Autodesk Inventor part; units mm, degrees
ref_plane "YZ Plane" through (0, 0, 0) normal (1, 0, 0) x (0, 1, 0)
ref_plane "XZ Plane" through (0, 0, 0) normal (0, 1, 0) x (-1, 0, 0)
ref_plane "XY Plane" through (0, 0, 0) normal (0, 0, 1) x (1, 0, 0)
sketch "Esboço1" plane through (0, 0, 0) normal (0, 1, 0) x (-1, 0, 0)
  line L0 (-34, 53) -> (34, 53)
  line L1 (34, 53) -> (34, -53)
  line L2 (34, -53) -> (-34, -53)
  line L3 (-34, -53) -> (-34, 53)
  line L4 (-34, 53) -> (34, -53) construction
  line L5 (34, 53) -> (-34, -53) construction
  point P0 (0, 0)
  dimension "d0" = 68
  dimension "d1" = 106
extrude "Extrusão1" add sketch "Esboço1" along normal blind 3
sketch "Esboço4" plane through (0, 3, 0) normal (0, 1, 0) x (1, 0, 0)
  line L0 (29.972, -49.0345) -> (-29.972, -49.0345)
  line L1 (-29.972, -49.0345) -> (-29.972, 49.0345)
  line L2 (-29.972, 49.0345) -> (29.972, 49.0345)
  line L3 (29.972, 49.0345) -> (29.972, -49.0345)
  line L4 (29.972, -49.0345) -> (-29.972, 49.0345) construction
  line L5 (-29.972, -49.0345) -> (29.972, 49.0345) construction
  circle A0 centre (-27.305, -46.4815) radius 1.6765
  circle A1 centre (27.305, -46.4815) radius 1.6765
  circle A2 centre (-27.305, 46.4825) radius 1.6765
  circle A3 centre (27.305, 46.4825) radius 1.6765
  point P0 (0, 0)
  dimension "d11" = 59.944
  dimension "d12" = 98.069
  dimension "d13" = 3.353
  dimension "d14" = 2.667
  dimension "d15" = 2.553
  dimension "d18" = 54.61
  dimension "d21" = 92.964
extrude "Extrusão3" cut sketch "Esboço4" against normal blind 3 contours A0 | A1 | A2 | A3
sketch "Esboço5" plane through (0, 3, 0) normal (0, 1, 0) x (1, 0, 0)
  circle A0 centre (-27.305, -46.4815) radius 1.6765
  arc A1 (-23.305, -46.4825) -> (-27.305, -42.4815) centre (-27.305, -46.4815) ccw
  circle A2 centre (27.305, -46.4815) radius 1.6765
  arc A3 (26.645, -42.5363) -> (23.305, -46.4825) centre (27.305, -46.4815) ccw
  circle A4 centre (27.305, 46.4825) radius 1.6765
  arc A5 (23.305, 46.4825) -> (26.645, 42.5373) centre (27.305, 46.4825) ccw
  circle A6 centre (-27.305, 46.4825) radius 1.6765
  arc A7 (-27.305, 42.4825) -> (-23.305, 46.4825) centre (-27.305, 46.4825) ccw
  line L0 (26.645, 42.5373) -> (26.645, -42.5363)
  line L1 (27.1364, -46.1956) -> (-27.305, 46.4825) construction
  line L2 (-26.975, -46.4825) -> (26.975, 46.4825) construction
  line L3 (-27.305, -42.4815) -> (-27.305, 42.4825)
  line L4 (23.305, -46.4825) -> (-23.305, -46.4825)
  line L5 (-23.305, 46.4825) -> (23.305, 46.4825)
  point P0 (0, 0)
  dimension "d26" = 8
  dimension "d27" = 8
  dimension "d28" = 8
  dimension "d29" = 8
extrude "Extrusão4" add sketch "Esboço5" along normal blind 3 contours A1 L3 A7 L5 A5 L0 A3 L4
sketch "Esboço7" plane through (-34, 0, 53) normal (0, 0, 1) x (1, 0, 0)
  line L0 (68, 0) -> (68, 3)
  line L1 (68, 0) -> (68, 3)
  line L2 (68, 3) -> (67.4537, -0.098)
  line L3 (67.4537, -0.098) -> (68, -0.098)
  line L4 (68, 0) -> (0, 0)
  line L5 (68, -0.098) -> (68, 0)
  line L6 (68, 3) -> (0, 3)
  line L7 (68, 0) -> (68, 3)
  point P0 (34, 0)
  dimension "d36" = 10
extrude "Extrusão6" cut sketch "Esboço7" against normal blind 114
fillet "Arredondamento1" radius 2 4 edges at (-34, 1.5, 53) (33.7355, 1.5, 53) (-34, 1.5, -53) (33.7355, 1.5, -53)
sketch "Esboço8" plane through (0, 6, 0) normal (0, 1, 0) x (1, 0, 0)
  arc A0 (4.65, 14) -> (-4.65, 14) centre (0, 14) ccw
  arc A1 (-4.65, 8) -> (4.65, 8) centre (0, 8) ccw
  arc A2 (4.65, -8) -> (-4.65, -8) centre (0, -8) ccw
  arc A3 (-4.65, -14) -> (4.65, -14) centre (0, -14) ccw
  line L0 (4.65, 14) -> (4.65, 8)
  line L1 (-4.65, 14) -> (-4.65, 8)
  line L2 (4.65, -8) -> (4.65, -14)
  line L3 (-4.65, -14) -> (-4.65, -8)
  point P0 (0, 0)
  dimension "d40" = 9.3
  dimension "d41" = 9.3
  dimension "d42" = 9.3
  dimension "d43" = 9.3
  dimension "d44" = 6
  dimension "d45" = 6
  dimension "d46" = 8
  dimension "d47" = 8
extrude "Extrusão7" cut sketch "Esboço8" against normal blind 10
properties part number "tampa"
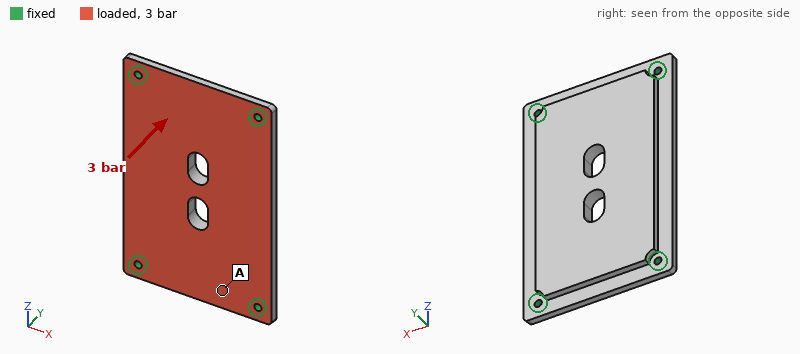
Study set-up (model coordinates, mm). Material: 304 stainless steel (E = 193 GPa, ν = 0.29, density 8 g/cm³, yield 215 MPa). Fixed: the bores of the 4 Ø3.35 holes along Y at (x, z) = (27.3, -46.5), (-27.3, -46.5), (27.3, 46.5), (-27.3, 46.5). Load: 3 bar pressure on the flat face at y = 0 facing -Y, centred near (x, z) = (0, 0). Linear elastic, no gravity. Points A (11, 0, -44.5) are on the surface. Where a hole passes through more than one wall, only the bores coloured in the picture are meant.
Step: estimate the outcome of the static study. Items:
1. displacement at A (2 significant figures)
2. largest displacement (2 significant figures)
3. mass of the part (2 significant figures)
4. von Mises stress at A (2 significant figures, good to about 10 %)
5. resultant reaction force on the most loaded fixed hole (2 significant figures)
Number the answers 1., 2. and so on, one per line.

1. 9.0 µm
2. 54 µm
3. 280 g
4. 13 MPa
5. 1.0 kN
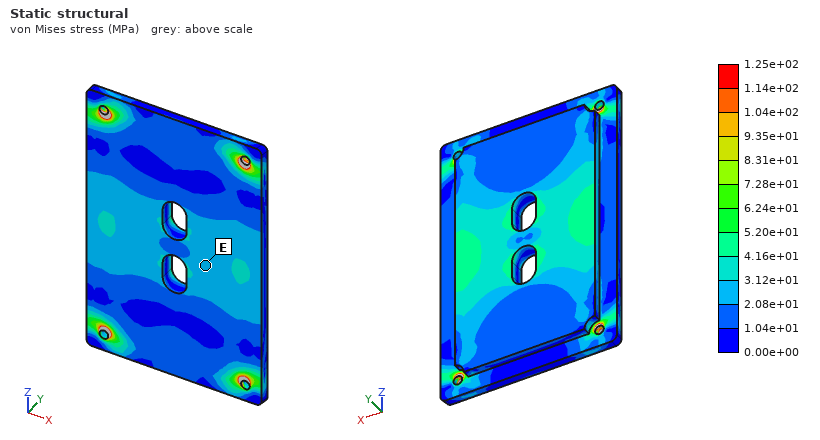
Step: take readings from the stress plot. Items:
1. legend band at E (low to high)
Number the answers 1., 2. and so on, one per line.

1. 2.08e+01 to 3.12e+01 MPa
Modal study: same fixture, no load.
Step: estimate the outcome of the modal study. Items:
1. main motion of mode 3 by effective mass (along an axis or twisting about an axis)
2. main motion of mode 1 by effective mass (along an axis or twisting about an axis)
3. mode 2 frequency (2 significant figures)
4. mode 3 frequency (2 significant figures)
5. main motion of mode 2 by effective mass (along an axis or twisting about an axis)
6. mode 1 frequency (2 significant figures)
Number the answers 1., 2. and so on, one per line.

1. twisting about X
2. along Y
3. 3700 Hz
4. 5600 Hz
5. twisting about Z
6. 2100 Hz
